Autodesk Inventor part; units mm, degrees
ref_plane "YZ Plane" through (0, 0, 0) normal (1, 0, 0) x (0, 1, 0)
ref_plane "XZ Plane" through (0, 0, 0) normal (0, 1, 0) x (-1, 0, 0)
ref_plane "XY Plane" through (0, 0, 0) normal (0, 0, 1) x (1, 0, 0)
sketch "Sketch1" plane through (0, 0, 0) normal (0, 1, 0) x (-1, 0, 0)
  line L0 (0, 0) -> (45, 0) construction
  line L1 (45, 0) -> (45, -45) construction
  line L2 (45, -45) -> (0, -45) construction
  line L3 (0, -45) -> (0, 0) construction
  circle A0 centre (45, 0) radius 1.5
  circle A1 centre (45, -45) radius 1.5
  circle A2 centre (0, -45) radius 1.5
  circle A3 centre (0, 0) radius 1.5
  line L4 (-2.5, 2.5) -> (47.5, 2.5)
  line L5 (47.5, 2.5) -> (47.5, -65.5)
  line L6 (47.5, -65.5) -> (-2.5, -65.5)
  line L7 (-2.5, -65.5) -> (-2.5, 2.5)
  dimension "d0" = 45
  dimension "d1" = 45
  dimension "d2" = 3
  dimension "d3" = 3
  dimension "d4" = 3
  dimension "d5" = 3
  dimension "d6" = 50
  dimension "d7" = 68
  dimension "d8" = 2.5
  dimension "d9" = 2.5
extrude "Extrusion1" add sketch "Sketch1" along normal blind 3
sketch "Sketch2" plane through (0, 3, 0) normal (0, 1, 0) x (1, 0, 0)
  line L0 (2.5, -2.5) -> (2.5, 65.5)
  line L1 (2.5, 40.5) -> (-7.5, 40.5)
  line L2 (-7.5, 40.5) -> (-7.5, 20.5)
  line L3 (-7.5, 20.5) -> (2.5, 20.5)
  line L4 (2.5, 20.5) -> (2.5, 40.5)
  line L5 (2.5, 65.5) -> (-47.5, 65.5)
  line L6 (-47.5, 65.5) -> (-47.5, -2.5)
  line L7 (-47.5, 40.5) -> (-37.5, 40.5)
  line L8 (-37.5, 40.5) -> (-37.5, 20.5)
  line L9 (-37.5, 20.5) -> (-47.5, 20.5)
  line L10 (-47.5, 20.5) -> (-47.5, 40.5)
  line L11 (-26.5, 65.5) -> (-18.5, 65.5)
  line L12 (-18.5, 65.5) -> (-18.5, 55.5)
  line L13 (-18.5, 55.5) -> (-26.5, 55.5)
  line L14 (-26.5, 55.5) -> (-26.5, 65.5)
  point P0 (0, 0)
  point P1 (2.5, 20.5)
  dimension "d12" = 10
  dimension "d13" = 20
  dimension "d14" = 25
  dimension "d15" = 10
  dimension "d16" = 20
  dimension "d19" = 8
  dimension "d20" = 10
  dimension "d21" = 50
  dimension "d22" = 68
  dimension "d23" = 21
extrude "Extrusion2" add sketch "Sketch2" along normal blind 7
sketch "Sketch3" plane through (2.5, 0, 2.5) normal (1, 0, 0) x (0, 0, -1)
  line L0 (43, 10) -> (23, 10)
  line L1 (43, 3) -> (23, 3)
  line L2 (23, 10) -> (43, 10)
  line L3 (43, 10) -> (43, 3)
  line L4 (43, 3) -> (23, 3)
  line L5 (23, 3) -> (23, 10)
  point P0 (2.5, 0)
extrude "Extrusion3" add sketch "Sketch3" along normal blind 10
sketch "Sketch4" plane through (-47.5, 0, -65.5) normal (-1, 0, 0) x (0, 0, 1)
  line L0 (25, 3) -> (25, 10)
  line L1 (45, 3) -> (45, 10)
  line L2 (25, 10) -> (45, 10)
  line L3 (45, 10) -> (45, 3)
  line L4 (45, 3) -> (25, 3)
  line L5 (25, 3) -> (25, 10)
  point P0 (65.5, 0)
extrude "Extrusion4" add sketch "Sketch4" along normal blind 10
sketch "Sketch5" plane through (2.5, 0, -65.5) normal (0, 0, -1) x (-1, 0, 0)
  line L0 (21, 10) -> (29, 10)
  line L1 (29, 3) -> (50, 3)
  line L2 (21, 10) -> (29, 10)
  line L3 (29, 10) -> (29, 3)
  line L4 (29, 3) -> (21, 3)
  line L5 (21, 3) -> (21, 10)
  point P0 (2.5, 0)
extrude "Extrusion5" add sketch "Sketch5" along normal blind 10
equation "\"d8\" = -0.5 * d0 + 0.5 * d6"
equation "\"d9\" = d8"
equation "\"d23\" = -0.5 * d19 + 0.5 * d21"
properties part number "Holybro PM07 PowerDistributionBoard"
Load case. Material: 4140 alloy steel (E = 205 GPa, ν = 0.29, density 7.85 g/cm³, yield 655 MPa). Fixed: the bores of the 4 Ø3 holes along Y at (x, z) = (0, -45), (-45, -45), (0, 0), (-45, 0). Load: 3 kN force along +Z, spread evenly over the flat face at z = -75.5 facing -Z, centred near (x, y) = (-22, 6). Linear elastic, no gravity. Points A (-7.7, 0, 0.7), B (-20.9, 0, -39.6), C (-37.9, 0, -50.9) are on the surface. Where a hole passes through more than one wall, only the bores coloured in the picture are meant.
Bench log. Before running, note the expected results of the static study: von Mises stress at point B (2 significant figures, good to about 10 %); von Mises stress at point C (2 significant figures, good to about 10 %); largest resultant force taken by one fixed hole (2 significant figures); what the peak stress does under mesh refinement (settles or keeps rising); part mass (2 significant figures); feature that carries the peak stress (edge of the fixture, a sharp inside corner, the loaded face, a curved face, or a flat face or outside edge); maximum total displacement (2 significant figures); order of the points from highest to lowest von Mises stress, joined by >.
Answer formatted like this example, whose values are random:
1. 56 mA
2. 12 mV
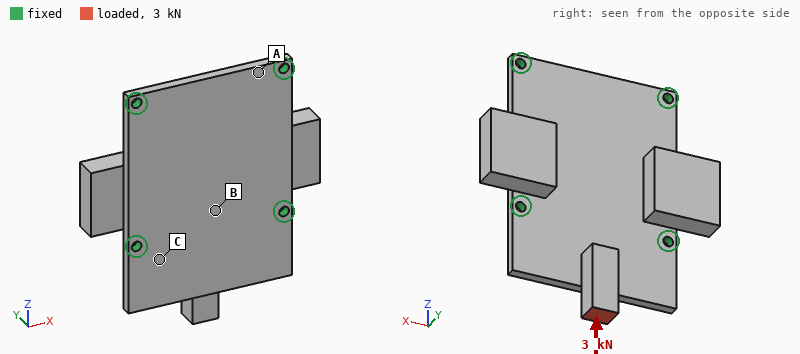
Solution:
1. 63 MPa
2. 170 MPa
3. 1.1 kN
4. keeps rising
5. 130 g
6. edge of the fixture
7. 0.35 mm
8. C > B > A
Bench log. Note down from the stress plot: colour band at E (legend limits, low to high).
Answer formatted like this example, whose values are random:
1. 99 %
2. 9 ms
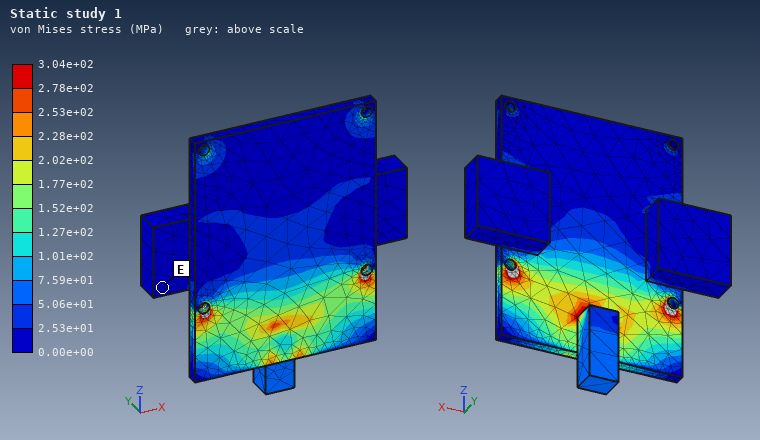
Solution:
1. 0.00e+00 to 2.53e+01 MPa
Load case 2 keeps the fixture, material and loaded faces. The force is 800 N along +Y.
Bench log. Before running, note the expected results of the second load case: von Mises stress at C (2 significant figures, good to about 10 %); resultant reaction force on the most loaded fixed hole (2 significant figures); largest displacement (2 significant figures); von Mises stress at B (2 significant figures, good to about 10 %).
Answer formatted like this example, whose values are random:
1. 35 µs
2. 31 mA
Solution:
1. 260 MPa
2. 560 N
3. 0.52 mm
4. 130 MPa
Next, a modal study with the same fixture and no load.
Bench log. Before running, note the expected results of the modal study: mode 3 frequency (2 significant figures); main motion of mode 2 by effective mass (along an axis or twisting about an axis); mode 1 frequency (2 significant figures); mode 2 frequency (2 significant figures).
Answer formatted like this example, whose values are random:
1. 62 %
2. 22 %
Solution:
1. 5100 Hz
2. along Y
3. 2500 Hz
4. 4600 Hz
